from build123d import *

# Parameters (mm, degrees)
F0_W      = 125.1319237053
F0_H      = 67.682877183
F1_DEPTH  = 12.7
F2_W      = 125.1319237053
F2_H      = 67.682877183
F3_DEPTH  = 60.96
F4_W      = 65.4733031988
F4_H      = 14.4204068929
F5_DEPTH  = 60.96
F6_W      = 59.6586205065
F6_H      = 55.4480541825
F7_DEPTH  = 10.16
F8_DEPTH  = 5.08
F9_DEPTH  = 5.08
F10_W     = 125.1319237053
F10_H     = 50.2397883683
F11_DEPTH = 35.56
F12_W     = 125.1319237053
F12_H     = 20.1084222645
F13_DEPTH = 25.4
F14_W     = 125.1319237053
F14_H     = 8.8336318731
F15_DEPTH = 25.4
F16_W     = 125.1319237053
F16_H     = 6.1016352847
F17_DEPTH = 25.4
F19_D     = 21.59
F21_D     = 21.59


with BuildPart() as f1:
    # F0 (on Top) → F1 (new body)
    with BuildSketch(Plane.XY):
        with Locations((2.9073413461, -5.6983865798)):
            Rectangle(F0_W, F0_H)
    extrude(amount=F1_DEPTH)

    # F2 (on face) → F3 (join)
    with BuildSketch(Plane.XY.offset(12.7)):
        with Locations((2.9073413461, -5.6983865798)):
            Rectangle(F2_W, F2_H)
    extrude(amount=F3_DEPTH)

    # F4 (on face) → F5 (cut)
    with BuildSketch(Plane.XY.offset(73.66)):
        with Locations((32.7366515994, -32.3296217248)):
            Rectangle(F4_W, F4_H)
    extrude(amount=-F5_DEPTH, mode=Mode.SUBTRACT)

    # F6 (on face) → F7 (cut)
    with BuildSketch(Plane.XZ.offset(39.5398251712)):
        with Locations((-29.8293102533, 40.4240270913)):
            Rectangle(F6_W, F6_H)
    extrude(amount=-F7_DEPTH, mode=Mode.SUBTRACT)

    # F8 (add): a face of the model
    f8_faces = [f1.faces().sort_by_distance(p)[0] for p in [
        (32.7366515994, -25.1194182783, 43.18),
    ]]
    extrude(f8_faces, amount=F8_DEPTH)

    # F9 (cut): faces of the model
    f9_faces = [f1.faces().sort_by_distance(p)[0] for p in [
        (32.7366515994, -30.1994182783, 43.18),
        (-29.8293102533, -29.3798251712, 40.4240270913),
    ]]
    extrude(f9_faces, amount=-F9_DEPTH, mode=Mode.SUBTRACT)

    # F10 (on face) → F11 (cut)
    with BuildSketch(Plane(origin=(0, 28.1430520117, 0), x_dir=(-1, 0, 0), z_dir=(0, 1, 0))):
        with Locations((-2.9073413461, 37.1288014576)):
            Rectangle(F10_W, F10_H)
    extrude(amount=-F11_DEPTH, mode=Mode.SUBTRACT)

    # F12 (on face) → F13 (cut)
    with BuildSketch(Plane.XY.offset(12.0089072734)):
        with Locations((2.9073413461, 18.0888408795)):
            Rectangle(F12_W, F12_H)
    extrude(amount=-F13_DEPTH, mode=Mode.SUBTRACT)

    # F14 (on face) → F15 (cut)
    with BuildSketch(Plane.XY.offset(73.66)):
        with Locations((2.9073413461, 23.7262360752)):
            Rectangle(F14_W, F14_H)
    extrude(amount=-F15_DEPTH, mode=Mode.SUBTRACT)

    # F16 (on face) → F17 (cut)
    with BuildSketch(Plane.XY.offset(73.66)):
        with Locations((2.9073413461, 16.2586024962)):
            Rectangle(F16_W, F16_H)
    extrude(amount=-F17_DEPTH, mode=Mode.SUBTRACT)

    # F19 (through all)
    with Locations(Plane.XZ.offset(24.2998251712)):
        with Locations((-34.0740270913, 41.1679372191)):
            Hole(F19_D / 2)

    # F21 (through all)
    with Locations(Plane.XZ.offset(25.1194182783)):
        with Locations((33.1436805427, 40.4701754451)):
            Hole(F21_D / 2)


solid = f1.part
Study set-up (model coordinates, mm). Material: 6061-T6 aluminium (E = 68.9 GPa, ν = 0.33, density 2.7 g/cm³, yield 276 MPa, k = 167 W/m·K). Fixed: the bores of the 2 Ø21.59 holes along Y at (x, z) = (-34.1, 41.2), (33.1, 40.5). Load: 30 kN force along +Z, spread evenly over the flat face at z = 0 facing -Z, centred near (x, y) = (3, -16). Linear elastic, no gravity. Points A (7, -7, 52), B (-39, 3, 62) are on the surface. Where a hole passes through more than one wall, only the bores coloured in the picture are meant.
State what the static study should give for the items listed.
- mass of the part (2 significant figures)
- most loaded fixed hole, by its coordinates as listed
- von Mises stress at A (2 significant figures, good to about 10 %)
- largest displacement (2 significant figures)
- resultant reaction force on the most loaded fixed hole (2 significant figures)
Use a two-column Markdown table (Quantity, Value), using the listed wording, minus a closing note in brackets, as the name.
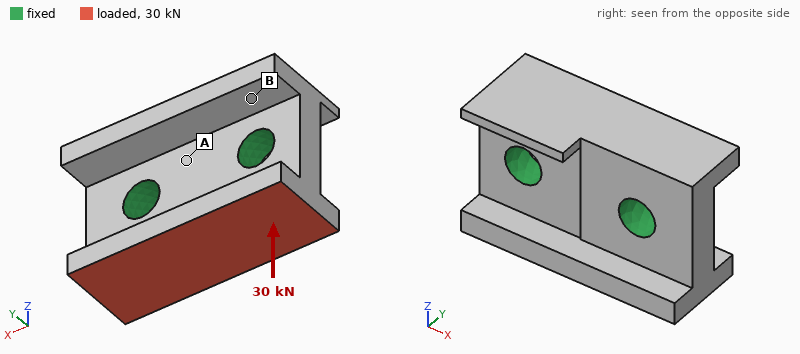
| Quantity | Value |
|---|---|
| mass of the part | 620 g |
| most loaded fixed hole, by its coordinates as listed | (33.1, 40.5) |
| von Mises stress at A | 5.1 MPa |
| largest displacement | 23 µm |
| resultant reaction force on the most loaded fixed hole | 16 kN |
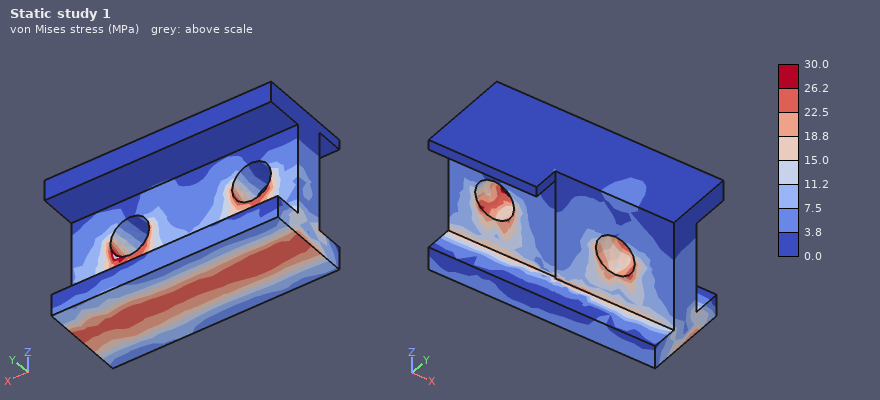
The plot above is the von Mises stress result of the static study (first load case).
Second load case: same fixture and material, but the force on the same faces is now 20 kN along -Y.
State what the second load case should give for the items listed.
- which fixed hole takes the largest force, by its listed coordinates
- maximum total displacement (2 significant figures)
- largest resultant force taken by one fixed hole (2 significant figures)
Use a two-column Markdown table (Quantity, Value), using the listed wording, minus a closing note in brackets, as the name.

| Quantity | Value |
|---|---|
| which fixed hole takes the largest force, by its listed coordinates | (33.1, 40.5) |
| maximum total displacement | 0.13 mm |
| largest resultant force taken by one fixed hole | 11 kN |
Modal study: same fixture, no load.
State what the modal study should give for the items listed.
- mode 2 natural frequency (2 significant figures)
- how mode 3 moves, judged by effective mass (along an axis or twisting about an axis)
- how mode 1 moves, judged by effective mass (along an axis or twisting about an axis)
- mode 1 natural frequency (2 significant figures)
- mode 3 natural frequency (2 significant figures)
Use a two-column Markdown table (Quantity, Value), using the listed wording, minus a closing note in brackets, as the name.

| Quantity | Value |
|---|---|
| mode 2 natural frequency | 6600 Hz |
| how mode 3 moves, judged by effective mass | along Y |
| how mode 1 moves, judged by effective mass | along Y |
| mode 1 natural frequency | 5500 Hz |
| mode 3 natural frequency | 7400 Hz |
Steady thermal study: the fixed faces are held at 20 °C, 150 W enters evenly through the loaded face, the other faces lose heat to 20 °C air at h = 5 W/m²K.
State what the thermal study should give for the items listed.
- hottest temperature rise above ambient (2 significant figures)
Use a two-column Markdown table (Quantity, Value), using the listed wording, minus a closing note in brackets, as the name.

| Quantity | Value |
|---|---|
| hottest temperature rise above ambient | 15 K |
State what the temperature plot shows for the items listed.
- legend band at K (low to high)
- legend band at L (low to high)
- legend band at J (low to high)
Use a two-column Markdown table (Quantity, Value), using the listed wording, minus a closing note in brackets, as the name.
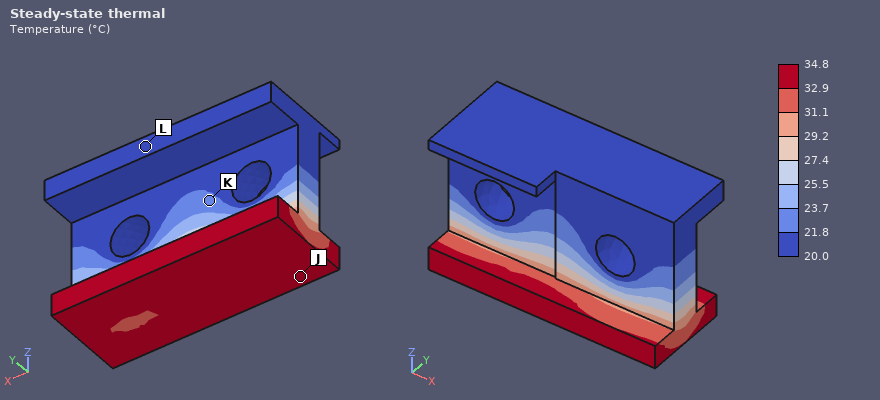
| Quantity | Value |
|---|---|
| legend band at K | 21.8 to 23.7 °C |
| legend band at L | 20.0 to 21.8 °C |
| legend band at J | 32.9 to 34.8 °C |
